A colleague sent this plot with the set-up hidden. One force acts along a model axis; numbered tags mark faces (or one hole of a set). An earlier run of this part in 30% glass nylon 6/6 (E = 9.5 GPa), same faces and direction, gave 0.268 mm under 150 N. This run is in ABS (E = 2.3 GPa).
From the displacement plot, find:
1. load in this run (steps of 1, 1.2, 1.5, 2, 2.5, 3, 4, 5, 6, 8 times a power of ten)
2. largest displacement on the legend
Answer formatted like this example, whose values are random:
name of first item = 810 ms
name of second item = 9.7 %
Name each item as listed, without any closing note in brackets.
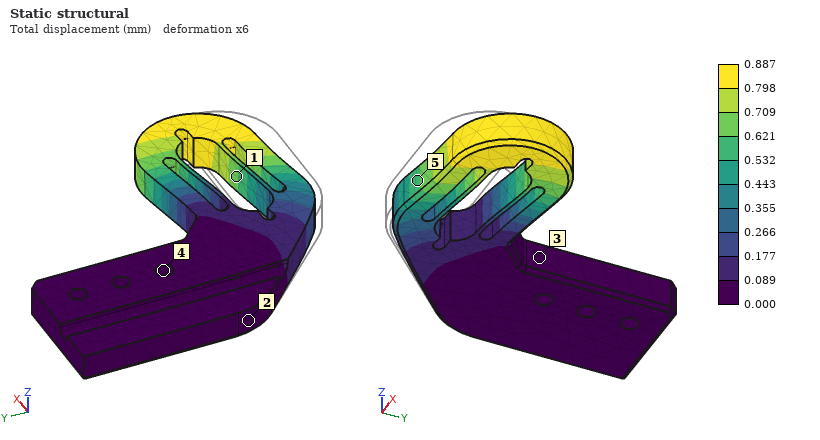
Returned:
load in this run = 120 N
largest displacement on the legend = 0.887 mm
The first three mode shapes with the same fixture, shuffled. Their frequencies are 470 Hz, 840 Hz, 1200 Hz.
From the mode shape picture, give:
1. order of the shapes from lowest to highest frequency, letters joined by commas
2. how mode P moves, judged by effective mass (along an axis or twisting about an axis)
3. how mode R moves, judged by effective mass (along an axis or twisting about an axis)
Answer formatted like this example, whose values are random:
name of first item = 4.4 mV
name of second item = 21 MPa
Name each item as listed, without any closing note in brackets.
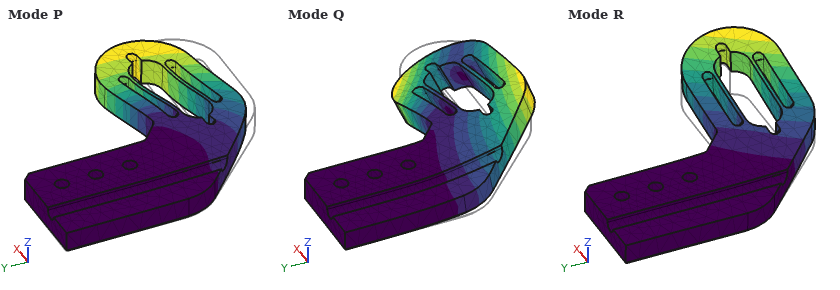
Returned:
order of the shapes from lowest to highest frequency, letters joined by commas = R, P, Q
how mode P moves, judged by effective mass = along Y
how mode R moves, judged by effective mass = along Z
